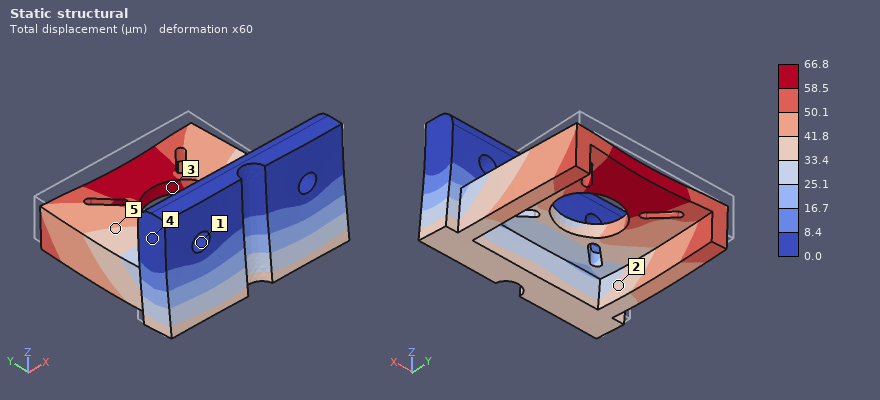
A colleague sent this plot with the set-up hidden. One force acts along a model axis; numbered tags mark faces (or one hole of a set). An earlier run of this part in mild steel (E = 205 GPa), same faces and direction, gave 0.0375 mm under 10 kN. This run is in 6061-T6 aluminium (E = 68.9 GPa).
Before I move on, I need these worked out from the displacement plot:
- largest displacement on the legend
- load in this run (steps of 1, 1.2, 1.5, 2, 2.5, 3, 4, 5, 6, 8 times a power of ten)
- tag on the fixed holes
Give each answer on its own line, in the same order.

66.8 µm
6 kN
1
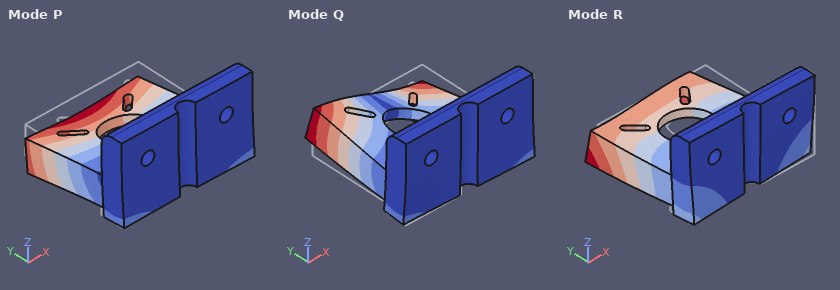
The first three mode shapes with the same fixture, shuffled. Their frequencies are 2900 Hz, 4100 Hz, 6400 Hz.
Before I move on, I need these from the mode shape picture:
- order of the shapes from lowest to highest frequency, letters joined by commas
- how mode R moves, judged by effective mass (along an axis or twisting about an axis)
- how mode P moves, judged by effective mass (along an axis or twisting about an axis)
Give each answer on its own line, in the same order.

P, Q, R
along X
along Z
